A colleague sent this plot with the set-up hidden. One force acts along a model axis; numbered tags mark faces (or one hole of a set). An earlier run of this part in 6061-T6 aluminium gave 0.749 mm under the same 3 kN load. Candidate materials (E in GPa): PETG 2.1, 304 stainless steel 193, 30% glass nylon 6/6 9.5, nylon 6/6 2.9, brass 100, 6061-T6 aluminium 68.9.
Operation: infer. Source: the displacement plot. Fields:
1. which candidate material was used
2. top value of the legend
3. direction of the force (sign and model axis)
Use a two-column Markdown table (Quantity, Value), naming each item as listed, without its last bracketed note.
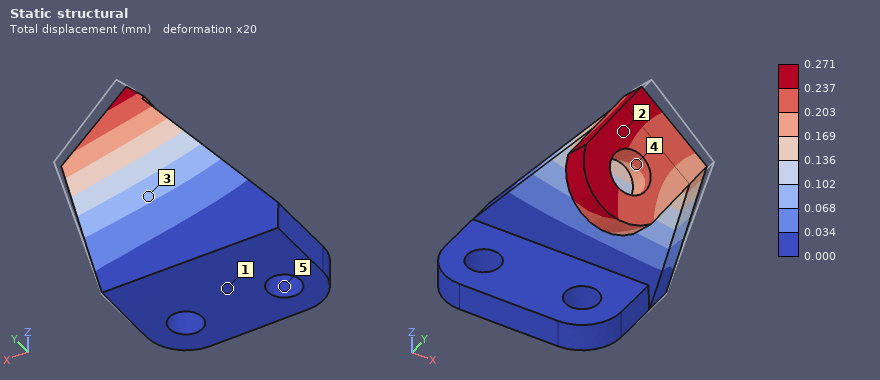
| Quantity | Value |
|---|---|
| which candidate material was used | 304 stainless steel |
| top value of the legend | 0.271 mm |
| direction of the force | -Y |
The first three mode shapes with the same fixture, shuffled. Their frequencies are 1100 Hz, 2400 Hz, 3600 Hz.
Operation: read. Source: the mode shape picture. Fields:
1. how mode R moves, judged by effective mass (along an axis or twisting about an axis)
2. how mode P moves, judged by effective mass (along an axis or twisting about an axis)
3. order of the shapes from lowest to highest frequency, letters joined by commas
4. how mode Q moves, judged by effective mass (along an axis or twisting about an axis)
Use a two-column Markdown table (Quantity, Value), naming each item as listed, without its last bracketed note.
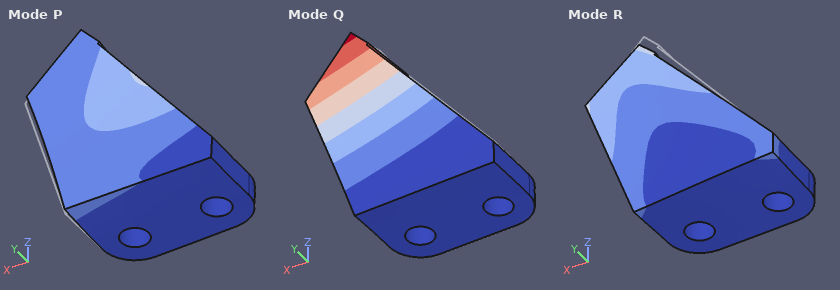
| Quantity | Value |
|---|---|
| how mode R moves, judged by effective mass | along X |
| how mode P moves, judged by effective mass | along Z |
| order of the shapes from lowest to highest frequency, letters joined by commas | Q, R, P |
| how mode Q moves, judged by effective mass | along Y |
